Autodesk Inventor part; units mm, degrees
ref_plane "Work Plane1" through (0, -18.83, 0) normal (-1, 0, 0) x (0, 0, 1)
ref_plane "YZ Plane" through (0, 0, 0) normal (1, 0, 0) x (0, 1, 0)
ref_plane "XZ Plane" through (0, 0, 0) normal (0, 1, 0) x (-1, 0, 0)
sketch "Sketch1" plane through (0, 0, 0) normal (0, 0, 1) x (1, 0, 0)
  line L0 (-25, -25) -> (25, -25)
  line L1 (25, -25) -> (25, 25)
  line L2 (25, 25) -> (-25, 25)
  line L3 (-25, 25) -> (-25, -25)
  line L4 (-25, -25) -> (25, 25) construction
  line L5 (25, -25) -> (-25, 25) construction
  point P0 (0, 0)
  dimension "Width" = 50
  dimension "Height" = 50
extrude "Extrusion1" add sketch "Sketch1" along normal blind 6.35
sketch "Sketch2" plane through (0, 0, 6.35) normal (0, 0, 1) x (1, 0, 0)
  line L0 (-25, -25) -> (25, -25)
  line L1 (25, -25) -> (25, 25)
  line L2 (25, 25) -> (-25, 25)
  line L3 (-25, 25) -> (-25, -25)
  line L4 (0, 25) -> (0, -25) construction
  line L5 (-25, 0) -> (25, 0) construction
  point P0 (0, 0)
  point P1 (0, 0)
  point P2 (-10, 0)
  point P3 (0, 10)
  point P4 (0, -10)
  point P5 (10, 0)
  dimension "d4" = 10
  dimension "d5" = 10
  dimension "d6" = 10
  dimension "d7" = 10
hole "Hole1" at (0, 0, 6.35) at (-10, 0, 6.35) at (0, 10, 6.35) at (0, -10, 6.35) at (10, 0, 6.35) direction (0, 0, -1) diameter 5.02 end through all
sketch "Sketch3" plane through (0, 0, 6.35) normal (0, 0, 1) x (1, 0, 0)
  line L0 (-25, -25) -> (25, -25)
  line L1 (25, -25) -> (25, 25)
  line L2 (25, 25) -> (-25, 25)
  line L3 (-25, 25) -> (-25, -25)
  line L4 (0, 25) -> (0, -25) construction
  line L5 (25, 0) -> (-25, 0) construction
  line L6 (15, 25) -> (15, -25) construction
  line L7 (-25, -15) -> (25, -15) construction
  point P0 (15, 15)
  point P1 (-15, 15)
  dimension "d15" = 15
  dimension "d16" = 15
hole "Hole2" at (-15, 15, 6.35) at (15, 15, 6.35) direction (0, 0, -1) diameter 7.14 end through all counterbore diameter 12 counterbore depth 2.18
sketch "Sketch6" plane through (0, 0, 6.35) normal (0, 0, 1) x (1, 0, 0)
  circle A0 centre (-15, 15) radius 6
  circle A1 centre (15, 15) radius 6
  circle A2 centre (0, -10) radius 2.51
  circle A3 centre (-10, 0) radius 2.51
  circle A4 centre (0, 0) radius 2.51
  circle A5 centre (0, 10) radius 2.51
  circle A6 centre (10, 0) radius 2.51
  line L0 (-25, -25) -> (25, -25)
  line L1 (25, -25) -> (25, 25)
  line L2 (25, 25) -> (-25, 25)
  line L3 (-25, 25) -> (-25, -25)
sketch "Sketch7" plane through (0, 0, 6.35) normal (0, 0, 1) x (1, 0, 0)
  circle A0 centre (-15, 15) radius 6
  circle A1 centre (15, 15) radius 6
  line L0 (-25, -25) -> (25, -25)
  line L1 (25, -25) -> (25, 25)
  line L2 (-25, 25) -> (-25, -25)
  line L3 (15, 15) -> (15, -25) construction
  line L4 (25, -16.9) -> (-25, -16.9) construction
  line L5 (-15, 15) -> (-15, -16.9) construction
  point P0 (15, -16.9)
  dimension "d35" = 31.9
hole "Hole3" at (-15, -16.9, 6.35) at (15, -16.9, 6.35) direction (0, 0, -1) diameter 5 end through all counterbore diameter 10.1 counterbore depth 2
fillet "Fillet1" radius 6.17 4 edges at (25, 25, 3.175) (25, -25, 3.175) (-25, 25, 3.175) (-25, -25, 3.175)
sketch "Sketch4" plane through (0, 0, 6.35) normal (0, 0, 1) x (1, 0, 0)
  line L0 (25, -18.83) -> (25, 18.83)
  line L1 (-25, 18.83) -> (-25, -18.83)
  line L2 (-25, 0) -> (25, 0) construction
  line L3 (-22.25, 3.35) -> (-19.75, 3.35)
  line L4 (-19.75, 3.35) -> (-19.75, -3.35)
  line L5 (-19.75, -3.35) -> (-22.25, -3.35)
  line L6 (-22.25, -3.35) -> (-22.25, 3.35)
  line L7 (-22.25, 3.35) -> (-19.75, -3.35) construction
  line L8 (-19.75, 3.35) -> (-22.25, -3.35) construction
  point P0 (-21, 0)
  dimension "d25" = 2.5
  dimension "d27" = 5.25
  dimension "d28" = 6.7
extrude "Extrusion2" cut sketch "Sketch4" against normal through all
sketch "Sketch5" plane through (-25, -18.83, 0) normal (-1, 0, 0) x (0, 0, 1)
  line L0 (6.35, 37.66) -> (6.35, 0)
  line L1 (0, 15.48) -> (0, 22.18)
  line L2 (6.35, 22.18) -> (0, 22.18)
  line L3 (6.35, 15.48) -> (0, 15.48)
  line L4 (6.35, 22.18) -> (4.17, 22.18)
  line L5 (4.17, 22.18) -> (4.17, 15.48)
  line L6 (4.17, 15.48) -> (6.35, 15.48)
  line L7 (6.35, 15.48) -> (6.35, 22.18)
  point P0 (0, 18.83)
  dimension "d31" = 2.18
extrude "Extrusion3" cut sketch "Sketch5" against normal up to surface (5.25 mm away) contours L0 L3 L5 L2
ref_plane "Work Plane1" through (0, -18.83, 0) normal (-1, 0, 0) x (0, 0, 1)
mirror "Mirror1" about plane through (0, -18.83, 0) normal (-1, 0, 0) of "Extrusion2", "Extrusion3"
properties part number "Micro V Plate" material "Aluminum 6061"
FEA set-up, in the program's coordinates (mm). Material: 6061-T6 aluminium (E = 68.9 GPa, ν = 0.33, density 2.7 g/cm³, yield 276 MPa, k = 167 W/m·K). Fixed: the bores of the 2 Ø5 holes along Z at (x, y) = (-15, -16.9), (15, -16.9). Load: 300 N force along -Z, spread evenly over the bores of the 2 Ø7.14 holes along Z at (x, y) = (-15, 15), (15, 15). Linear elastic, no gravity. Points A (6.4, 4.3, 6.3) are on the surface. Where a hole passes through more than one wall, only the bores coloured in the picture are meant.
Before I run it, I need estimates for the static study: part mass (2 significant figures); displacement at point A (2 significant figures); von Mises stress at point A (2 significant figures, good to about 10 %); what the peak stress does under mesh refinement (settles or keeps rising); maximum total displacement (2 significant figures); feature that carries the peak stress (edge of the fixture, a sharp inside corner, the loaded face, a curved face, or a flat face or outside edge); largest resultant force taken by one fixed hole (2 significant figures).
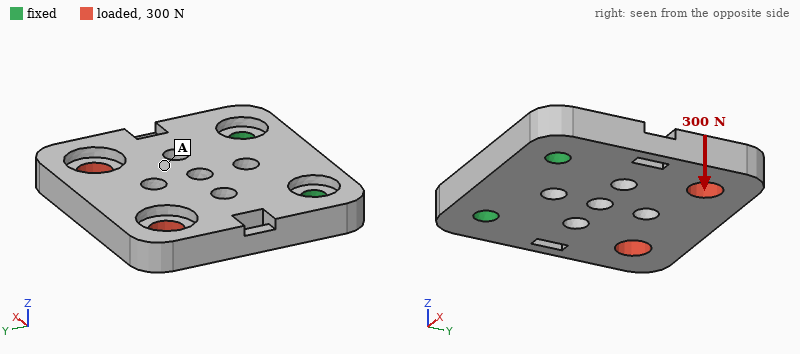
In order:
36 g
0.044 mm
13 MPa
keeps rising
0.11 mm
edge of the fixture
150 N
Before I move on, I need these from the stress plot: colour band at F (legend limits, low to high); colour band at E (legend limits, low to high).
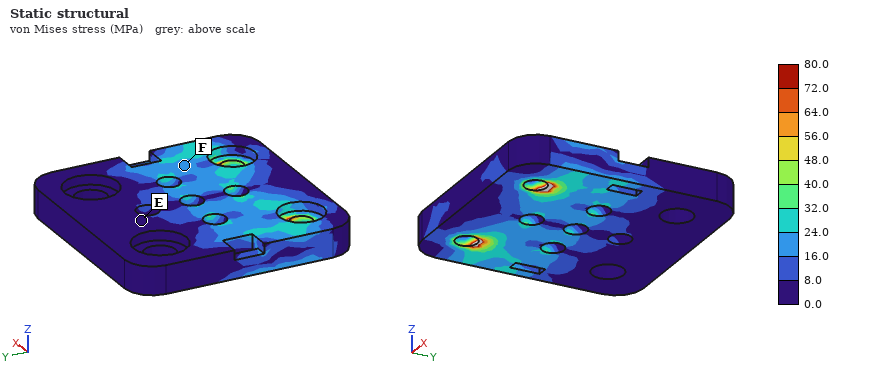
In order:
16.0 to 24.0 MPa
0.0 to 8.0 MPa
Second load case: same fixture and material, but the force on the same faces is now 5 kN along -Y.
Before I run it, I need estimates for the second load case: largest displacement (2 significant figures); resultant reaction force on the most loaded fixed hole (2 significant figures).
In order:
63 µm
2.5 kN
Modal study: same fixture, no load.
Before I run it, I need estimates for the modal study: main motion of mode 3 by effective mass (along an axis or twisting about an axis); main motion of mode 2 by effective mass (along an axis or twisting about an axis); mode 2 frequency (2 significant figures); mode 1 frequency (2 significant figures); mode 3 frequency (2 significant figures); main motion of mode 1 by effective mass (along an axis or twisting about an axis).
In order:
along X
twisting about Y
5400 Hz
2400 Hz
11 kHz
along Z
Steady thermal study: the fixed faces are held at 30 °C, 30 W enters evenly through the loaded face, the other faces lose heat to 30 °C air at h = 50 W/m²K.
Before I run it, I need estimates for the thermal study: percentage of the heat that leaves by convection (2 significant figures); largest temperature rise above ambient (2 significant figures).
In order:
13 %
25 K
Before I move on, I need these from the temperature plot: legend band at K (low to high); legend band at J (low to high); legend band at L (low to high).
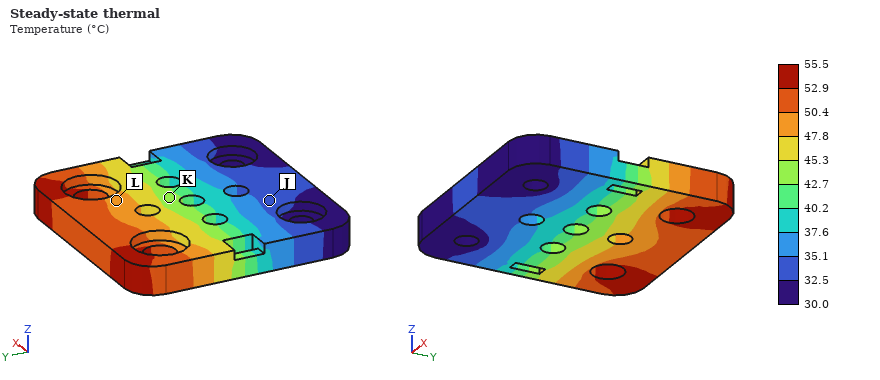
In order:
42.7 to 45.3 °C
32.5 to 35.1 °C
47.8 to 50.4 °C
